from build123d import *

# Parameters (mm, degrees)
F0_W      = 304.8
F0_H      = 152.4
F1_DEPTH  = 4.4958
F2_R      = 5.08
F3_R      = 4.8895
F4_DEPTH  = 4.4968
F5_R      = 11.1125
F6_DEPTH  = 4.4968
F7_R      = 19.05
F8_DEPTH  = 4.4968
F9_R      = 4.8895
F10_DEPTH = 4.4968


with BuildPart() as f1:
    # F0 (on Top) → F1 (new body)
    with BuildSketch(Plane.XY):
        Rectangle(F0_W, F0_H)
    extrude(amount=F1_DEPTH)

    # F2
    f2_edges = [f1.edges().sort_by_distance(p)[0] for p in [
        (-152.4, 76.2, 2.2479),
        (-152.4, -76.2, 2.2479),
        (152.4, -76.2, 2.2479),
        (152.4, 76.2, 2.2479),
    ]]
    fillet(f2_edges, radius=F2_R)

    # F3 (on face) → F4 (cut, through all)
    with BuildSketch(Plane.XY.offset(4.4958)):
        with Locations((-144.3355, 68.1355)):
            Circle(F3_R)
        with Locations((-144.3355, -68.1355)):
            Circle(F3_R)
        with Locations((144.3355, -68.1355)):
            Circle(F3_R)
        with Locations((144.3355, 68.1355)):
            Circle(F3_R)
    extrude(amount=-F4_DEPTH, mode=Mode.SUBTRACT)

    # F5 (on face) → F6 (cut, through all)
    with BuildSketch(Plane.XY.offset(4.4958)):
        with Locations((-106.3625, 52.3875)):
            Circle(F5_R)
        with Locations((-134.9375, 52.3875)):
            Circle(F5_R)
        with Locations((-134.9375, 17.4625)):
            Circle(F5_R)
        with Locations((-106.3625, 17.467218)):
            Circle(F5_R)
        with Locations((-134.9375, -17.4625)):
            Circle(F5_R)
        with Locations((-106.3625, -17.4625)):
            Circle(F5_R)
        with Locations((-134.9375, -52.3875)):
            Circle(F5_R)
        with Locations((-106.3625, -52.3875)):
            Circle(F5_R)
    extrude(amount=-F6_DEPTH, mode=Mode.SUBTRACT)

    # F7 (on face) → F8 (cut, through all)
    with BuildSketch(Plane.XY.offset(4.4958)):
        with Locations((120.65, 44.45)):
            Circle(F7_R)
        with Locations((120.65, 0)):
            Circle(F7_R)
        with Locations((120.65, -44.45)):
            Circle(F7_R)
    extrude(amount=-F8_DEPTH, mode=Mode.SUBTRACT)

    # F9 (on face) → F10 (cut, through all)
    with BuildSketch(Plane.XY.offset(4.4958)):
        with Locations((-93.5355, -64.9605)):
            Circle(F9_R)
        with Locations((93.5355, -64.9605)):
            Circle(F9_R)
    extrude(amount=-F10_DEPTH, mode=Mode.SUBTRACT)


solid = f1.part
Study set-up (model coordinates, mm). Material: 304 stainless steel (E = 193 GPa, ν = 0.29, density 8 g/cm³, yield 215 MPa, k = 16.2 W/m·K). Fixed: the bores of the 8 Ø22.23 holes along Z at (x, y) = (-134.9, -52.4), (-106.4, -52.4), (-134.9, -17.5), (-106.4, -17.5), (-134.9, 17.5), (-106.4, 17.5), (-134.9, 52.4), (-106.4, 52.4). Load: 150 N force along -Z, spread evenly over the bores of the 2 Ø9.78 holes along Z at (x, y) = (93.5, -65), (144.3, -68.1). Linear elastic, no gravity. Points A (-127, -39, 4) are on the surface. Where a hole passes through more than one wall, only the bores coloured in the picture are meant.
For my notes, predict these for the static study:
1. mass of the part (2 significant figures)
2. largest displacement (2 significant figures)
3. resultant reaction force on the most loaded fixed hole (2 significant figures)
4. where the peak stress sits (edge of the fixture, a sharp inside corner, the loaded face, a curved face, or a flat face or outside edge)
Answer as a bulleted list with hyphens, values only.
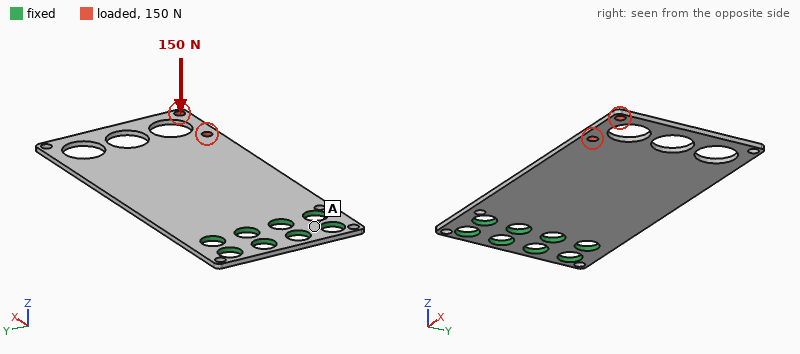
- 1.4 kg
- 3.2 mm
- 91 N
- a curved face
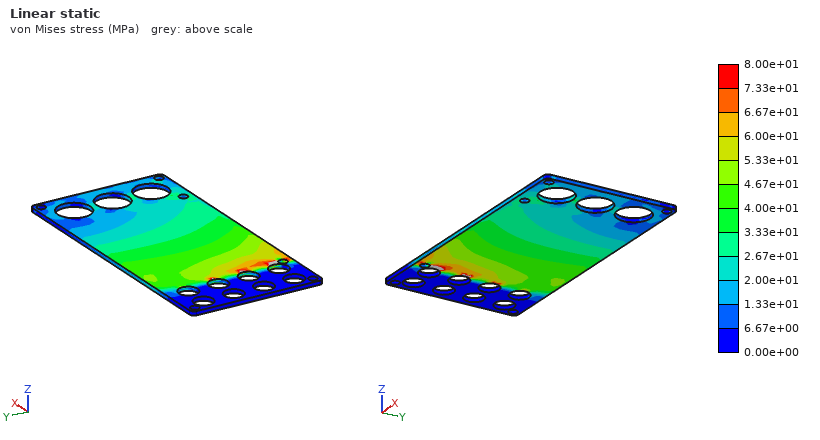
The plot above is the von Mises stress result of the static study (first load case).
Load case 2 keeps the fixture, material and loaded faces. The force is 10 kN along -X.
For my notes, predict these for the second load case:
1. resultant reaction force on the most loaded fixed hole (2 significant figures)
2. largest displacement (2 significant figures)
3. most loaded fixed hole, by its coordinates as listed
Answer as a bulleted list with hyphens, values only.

- 7.5 kN
- 0.13 mm
- (-106.4, -52.4)
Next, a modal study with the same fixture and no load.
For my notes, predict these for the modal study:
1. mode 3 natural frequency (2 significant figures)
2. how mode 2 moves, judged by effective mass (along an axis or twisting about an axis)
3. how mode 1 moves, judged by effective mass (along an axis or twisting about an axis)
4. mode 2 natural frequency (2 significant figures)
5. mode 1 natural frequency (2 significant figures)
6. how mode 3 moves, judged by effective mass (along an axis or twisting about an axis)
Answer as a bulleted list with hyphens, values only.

- 370 Hz
- twisting about X
- along Z
- 230 Hz
- 68 Hz
- along Z
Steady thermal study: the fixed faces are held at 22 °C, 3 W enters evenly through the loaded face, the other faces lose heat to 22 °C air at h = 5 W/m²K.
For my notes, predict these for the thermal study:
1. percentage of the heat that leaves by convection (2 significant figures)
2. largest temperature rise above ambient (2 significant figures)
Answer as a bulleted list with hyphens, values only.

- 88 %
- 57 K
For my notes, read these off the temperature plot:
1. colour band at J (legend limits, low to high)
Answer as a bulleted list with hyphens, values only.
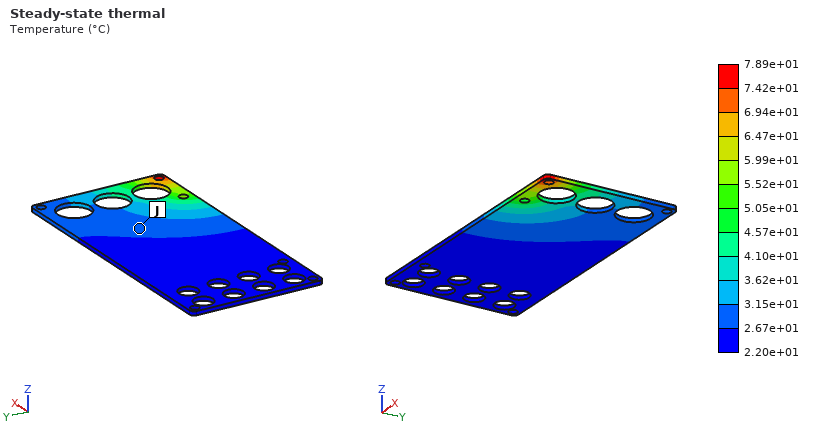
- 2.67e+01 to 3.15e+01 °C
